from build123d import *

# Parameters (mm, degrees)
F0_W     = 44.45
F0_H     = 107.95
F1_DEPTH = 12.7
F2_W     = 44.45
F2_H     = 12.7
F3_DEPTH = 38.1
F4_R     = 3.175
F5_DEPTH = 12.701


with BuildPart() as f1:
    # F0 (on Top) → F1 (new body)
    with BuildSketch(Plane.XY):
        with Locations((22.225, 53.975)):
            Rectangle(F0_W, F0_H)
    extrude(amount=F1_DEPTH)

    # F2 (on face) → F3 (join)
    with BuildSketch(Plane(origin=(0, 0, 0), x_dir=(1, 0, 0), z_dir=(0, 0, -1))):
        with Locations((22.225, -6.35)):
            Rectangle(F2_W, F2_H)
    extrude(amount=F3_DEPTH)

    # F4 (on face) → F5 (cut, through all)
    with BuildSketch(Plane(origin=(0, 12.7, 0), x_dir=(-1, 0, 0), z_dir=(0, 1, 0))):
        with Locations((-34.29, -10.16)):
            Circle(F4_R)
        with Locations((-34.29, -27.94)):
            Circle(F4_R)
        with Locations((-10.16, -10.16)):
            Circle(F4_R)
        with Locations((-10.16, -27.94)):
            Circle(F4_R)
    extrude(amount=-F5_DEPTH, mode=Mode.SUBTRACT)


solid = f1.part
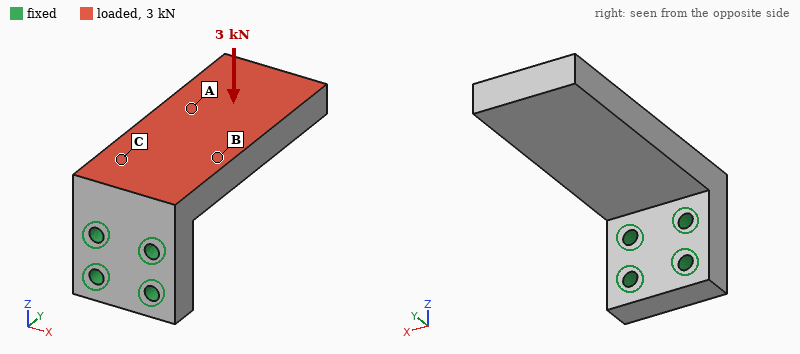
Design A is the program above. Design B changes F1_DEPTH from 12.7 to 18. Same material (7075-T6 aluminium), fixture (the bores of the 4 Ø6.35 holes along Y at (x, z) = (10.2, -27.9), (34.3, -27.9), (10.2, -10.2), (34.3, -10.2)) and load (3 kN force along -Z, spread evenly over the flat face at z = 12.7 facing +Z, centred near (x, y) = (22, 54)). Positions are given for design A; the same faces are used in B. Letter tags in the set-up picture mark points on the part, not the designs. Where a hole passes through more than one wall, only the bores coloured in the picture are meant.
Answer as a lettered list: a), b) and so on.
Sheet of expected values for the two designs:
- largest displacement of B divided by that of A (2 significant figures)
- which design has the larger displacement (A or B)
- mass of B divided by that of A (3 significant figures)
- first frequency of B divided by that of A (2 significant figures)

a) 0.63
b) A
c) 1.31
d) 1.0
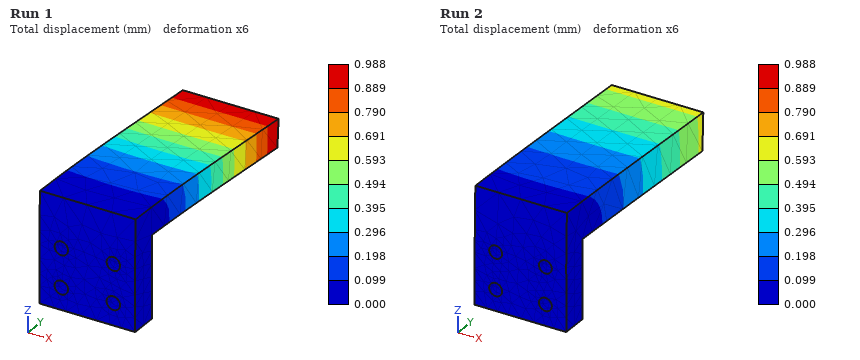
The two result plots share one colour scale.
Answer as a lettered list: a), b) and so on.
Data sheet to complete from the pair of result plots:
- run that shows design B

a) Run 2
